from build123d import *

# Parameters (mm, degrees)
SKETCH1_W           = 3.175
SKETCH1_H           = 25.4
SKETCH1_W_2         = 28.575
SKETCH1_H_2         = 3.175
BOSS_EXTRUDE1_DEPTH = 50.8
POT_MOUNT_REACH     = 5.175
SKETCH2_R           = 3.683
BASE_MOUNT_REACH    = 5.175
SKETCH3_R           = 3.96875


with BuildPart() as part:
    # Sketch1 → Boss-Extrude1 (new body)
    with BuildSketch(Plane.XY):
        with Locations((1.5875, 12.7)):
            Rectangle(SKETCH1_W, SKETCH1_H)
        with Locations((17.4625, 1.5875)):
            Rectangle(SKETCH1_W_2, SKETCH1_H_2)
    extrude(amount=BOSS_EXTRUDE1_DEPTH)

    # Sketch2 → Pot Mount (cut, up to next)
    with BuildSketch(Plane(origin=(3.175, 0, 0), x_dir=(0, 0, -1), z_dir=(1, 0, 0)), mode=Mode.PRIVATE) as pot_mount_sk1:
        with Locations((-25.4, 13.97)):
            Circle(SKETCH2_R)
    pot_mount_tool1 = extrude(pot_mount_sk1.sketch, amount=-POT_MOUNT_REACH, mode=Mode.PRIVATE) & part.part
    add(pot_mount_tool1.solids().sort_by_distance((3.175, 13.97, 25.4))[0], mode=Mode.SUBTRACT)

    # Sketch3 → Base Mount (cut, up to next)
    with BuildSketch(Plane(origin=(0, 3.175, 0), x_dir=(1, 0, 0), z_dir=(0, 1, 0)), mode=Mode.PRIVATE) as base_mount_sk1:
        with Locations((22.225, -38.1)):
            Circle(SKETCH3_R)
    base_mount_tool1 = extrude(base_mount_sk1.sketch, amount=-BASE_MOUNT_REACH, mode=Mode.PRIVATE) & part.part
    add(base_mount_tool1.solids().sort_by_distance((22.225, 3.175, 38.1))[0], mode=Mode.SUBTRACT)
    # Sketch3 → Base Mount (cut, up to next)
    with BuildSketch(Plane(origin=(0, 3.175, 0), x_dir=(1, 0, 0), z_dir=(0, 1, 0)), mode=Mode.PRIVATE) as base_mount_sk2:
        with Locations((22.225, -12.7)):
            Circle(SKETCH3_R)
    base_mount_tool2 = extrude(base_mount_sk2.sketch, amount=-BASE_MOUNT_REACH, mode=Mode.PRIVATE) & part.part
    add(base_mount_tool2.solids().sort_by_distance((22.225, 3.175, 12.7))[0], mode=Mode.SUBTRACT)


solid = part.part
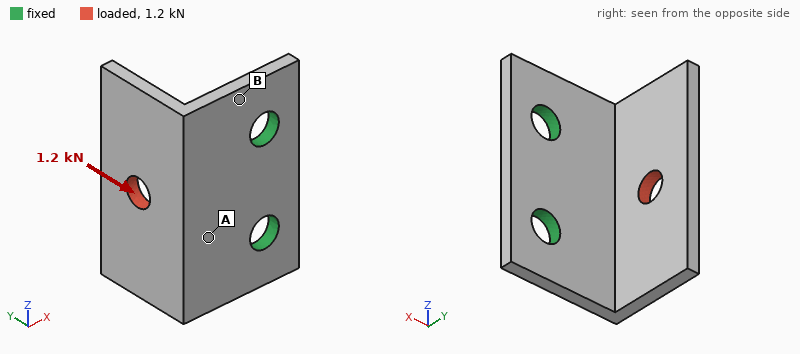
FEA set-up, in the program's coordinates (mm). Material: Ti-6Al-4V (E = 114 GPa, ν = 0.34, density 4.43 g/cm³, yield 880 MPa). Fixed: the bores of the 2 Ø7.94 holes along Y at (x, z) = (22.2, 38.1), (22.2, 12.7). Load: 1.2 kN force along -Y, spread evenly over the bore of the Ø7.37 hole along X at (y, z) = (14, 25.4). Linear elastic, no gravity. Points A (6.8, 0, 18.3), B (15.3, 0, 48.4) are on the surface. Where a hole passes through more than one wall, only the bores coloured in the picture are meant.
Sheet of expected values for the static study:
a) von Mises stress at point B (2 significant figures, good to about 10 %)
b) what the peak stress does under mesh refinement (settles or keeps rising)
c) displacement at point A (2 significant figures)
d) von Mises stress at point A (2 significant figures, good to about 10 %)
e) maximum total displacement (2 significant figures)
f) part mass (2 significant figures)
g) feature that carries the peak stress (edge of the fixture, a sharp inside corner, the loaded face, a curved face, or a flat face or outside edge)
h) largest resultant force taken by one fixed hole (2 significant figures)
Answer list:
140 MPa
keeps rising
0.097 mm
66 MPa
0.34 mm
37 g
edge of the fixture
600 N
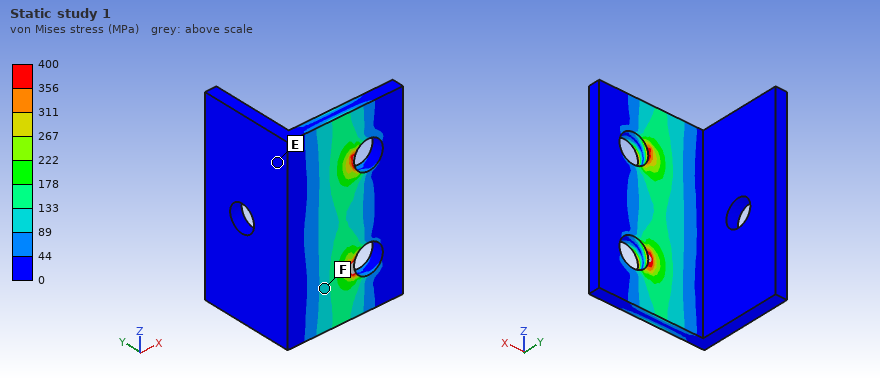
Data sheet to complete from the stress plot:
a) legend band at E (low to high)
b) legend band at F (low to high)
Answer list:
0 to 44 MPa
89 to 133 MPa
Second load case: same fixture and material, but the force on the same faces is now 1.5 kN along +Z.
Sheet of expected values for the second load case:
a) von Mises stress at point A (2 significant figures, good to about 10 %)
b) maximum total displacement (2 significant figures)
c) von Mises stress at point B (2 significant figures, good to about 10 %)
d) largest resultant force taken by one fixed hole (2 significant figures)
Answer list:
55 MPa
0.19 mm
96 MPa
1.3 kN
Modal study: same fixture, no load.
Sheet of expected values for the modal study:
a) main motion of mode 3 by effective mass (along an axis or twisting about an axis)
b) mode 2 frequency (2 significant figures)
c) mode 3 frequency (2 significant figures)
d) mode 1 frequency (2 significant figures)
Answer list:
along Y
3300 Hz
5500 Hz
2000 Hz
